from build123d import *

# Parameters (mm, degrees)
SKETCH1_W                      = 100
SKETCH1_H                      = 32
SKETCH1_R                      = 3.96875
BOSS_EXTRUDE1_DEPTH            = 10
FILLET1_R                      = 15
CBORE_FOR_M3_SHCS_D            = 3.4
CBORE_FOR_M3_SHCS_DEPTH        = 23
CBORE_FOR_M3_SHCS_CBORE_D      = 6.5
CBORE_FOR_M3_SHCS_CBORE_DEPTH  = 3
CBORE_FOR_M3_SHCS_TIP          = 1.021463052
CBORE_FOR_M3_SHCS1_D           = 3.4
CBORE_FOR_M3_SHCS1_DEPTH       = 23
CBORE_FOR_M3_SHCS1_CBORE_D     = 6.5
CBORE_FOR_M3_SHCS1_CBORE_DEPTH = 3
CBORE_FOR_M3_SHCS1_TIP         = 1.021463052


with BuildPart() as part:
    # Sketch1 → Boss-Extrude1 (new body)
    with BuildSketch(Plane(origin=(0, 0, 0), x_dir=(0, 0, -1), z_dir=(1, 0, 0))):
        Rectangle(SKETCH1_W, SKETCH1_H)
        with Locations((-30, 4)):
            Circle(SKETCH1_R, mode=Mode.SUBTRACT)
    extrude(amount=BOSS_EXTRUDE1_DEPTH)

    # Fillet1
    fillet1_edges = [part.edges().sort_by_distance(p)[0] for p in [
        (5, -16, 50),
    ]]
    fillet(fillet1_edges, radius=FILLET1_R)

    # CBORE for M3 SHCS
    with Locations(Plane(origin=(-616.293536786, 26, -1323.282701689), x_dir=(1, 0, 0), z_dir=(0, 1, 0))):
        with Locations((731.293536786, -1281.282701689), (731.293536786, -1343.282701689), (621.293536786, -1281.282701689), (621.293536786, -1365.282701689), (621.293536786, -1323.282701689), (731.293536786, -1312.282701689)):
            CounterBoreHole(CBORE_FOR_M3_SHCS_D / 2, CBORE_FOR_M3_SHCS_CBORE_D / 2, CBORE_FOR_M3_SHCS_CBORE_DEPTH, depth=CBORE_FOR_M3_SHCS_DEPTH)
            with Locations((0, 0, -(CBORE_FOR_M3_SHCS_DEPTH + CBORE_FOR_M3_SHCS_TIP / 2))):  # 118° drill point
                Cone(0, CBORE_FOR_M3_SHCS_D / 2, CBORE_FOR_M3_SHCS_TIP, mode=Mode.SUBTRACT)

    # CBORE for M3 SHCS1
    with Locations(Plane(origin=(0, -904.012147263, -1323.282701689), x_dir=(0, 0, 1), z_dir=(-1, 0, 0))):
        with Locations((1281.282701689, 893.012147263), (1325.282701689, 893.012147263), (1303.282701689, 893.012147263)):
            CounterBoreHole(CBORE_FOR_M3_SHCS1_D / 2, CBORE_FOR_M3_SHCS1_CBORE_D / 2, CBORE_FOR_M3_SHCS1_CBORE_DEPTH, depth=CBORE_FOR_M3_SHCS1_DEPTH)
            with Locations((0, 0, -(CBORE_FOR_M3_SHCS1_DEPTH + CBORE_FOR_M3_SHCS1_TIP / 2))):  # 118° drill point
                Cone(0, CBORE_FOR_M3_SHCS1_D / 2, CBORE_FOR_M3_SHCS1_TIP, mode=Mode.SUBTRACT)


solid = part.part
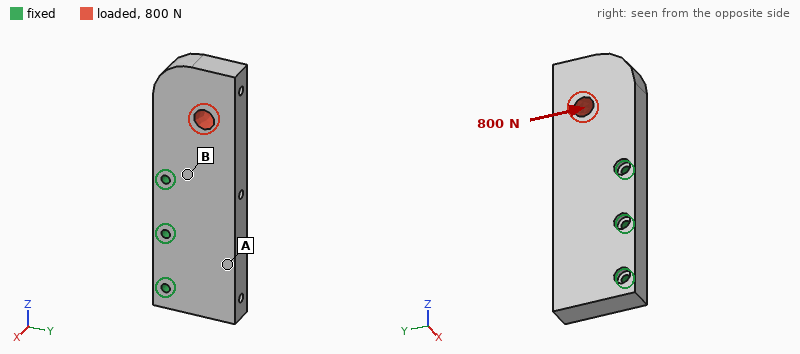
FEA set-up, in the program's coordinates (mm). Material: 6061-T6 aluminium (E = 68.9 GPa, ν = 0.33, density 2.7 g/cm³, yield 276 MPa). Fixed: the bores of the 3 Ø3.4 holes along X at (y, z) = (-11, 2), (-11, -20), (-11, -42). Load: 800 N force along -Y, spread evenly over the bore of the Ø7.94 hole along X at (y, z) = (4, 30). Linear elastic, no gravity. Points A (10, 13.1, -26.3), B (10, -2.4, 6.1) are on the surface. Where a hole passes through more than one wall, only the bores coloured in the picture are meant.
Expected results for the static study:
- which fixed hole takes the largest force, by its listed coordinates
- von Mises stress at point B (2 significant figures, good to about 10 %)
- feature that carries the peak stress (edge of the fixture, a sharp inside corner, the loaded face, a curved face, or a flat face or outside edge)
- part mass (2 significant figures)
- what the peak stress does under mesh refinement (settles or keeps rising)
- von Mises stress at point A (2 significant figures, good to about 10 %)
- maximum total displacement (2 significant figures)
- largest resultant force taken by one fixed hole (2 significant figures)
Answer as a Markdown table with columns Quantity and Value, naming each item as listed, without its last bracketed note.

| Quantity | Value |
|---|---|
| which fixed hole takes the largest force, by its listed coordinates | (-11, 2) |
| von Mises stress at point B | 8.7 MPa |
| feature that carries the peak stress | edge of the fixture |
| part mass | 81 g |
| what the peak stress does under mesh refinement | keeps rising |
| von Mises stress at point A | 3.4 MPa |
| maximum total displacement | 24 µm |
| largest resultant force taken by one fixed hole | 1.4 kN |
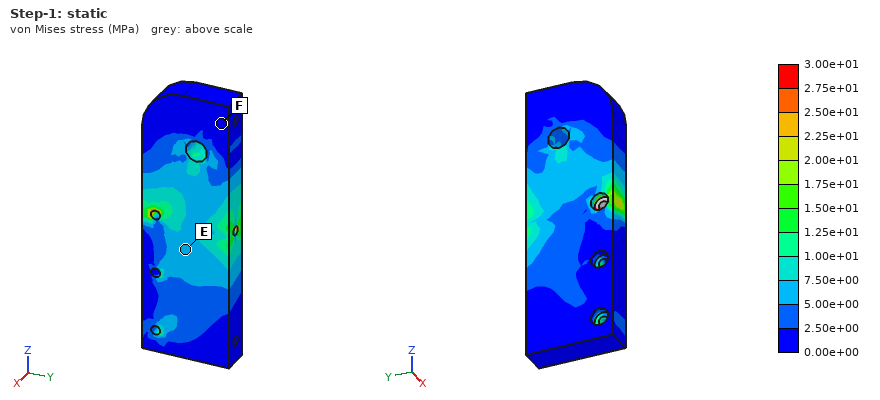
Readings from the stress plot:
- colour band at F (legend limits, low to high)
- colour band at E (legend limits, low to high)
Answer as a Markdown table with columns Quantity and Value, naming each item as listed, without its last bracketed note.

| Quantity | Value |
|---|---|
| colour band at F | 0.00e+00 to 2.50e+00 MPa |
| colour band at E | 5.00e+00 to 7.50e+00 MPa |
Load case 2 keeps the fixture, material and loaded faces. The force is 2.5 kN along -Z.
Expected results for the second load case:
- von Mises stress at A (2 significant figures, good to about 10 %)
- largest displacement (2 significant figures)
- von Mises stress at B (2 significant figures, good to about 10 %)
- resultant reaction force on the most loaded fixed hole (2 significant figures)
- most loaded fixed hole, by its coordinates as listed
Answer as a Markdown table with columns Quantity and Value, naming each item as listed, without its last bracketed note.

| Quantity | Value |
|---|---|
| von Mises stress at A | 4.3 MPa |
| largest displacement | 25 µm |
| von Mises stress at B | 8.3 MPa |
| resultant reaction force on the most loaded fixed hole | 1.4 kN |
| most loaded fixed hole, by its coordinates as listed | (-11, 2) |
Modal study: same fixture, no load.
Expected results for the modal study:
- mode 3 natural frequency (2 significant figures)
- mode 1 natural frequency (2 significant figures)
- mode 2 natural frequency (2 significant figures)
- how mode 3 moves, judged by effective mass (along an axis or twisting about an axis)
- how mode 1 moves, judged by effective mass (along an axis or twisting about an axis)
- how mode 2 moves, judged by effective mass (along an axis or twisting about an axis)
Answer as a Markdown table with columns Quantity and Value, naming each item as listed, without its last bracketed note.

| Quantity | Value |
|---|---|
| mode 3 natural frequency | 6300 Hz |
| mode 1 natural frequency | 2600 Hz |
| mode 2 natural frequency | 5800 Hz |
| how mode 3 moves, judged by effective mass | along Y |
| how mode 1 moves, judged by effective mass | along X |
| how mode 2 moves, judged by effective mass | along X |
